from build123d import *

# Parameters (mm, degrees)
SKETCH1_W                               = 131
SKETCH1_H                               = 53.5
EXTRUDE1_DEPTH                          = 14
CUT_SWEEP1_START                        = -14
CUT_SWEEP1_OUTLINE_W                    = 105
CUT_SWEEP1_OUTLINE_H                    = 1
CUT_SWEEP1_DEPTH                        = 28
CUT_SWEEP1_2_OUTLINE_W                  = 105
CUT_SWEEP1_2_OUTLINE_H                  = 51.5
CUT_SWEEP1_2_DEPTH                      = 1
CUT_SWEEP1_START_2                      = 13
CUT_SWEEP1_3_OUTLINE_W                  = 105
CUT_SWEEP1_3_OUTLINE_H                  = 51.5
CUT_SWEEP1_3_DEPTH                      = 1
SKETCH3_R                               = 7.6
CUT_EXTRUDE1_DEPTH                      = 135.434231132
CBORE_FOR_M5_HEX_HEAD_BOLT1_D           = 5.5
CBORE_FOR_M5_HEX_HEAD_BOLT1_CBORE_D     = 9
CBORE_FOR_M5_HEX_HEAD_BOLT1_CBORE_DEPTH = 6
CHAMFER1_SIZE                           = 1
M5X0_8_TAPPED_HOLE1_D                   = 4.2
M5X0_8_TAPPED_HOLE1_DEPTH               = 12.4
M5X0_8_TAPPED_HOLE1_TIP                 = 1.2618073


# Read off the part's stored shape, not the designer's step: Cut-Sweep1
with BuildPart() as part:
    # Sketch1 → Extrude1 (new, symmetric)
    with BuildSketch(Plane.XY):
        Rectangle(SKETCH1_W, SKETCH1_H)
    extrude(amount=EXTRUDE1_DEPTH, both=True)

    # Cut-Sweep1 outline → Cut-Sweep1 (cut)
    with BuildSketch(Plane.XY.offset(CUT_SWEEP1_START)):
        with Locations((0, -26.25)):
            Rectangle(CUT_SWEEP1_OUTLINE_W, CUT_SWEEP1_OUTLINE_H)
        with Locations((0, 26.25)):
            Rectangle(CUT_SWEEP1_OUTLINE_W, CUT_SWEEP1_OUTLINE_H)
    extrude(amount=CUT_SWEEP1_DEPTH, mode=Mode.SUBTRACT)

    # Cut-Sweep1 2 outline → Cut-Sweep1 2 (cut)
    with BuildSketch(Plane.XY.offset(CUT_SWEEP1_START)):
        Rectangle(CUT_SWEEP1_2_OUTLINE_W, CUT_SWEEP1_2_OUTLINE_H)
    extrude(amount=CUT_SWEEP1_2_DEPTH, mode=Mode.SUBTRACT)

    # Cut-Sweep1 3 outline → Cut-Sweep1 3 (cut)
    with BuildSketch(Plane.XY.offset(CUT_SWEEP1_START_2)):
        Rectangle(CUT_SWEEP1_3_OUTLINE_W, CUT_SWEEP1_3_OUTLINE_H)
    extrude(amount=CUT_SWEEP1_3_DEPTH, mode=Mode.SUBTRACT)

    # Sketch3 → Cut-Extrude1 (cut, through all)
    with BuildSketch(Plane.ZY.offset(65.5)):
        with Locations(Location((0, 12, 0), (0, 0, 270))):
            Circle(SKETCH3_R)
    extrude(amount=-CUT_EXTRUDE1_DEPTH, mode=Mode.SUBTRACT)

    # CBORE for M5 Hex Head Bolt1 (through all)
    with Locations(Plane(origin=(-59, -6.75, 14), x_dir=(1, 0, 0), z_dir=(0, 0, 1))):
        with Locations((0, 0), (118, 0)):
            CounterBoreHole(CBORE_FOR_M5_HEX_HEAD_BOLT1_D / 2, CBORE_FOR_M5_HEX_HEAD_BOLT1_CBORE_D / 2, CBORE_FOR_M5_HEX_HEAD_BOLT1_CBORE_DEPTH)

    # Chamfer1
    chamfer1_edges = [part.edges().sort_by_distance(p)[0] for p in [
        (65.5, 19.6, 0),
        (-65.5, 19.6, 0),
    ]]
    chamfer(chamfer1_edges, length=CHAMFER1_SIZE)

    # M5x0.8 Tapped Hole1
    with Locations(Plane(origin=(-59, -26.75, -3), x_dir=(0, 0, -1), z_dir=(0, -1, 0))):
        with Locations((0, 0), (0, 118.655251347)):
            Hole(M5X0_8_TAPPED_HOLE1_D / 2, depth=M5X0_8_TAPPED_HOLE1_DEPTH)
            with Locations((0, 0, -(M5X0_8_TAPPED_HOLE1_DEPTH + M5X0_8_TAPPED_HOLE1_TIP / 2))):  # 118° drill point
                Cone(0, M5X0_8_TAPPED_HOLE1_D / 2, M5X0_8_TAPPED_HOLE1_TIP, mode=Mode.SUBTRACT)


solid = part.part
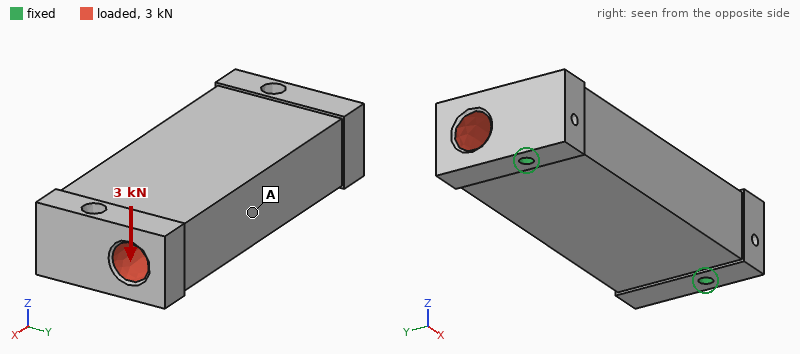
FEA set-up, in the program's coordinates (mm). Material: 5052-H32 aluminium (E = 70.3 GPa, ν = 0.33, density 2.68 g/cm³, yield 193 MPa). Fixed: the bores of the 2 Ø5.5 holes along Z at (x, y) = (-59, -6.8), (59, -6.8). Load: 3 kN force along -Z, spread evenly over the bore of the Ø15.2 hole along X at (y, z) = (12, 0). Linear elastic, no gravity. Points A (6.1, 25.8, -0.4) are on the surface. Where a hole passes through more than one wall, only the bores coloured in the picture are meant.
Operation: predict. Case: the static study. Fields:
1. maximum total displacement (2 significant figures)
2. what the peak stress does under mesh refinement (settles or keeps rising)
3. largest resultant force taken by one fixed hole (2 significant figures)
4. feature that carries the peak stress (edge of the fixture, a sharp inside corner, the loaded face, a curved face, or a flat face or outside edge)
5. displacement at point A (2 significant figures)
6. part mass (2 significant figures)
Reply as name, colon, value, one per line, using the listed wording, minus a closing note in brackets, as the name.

maximum total displacement: 18 µm
what the peak stress does under mesh refinement: keeps rising
largest resultant force taken by one fixed hole: 1.5 kN
feature that carries the peak stress: edge of the fixture
displacement at point A: 18 µm
part mass: 410 g
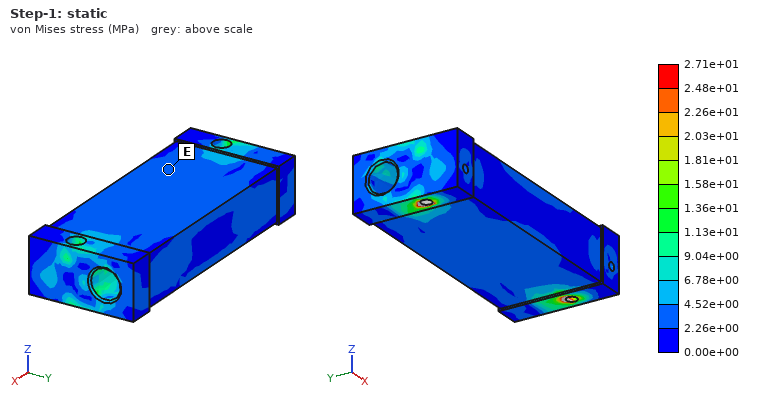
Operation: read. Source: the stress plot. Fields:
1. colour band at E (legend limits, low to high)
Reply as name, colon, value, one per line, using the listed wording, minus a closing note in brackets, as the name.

colour band at E: 2.26e+00 to 4.52e+00 MPa
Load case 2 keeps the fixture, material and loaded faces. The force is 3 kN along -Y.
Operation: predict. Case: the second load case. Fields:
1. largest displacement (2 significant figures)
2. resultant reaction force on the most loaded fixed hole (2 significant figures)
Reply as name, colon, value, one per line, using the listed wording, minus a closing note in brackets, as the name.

largest displacement: 5.2 µm
resultant reaction force on the most loaded fixed hole: 1.5 kN
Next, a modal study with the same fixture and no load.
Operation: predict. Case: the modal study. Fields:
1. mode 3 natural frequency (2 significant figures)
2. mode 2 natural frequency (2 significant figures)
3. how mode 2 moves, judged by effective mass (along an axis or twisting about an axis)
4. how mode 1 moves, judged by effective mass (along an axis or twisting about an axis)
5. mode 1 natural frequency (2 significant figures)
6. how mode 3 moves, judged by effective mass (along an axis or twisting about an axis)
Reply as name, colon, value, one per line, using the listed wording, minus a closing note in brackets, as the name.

mode 3 natural frequency: 7300 Hz
mode 2 natural frequency: 6800 Hz
how mode 2 moves, judged by effective mass: along Y
how mode 1 moves, judged by effective mass: along Z
mode 1 natural frequency: 5300 Hz
how mode 3 moves, judged by effective mass: along Y
